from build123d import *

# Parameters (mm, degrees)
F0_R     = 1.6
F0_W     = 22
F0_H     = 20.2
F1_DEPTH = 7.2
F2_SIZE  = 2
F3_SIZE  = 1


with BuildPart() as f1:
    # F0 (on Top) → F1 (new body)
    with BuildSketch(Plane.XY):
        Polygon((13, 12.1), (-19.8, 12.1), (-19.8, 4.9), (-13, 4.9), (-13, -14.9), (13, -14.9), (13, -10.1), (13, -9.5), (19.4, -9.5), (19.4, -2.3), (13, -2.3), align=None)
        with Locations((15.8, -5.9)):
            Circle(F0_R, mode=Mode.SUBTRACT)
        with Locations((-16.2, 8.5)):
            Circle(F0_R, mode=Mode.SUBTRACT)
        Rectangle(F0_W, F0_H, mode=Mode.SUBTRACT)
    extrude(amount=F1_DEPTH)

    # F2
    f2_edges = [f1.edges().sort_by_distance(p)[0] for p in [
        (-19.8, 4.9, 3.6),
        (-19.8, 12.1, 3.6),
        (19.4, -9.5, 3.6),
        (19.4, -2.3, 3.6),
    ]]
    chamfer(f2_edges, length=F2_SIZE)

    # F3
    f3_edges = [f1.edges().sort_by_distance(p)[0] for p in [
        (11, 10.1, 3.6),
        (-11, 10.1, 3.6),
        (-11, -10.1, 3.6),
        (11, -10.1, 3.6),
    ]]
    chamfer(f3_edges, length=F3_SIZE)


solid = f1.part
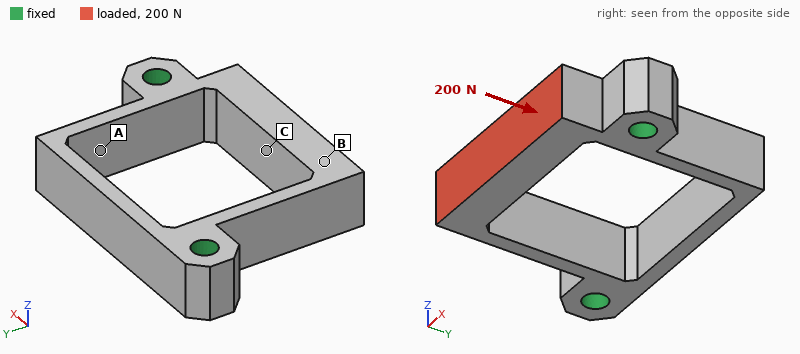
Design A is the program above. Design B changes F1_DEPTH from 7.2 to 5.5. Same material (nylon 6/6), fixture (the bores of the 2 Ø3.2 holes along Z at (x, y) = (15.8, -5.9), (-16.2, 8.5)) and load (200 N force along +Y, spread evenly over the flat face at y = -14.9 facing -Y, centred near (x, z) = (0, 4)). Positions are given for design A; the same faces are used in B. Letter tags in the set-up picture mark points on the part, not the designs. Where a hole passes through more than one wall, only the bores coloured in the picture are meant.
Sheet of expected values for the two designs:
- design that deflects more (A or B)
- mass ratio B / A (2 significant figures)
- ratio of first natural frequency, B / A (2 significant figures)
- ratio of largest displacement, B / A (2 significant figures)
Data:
B
0.76
0.82
1.3
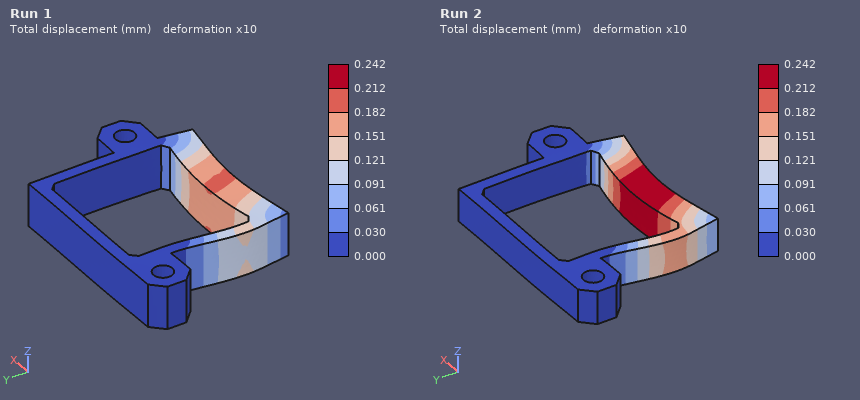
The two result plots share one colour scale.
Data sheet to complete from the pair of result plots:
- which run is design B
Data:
Run 2
